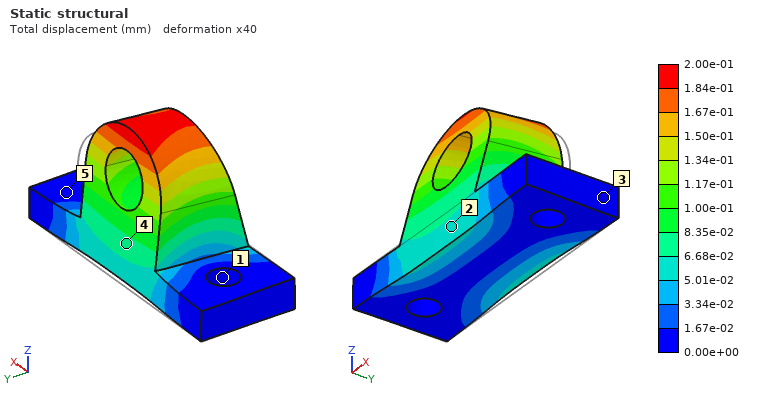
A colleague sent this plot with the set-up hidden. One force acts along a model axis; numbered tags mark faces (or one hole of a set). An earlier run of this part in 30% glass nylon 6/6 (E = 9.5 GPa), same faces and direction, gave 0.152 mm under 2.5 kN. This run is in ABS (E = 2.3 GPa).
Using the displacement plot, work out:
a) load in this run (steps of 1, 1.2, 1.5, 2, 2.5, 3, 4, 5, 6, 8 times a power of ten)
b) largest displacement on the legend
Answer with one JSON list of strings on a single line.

["800 N", "2.00e-01 mm"]
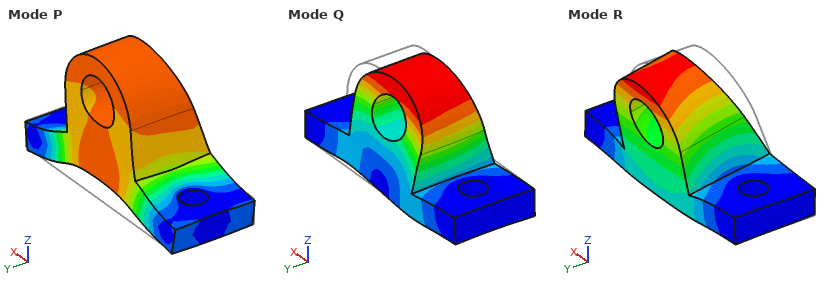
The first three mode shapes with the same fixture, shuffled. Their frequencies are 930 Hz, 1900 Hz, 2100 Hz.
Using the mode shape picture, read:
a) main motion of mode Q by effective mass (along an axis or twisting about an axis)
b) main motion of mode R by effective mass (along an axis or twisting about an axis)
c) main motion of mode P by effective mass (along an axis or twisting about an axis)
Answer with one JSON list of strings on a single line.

["along X", "along Y", "along Z"]
